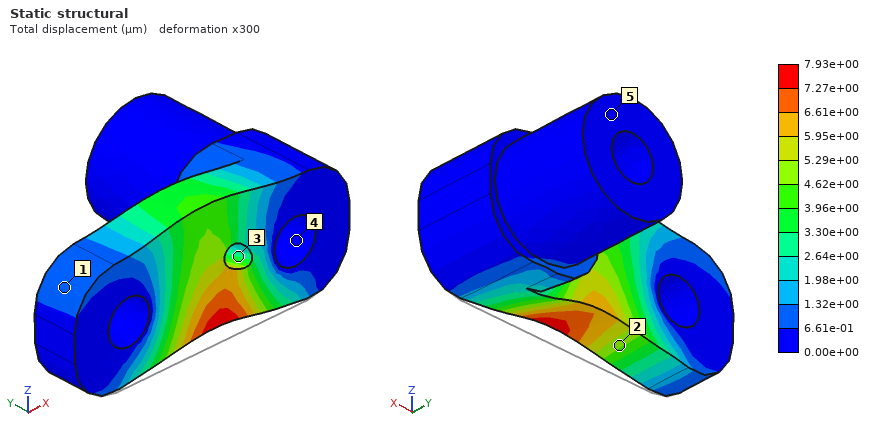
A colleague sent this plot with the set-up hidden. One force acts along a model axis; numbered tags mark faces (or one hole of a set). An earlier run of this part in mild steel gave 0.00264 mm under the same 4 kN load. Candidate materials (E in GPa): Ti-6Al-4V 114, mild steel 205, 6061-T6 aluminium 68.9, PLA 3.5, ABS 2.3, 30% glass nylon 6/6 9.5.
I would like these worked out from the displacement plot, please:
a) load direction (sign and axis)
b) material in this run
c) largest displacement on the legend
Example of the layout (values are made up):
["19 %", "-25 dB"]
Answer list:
["+Z", "6061-T6 aluminium", "7.93e+00 µm"]
